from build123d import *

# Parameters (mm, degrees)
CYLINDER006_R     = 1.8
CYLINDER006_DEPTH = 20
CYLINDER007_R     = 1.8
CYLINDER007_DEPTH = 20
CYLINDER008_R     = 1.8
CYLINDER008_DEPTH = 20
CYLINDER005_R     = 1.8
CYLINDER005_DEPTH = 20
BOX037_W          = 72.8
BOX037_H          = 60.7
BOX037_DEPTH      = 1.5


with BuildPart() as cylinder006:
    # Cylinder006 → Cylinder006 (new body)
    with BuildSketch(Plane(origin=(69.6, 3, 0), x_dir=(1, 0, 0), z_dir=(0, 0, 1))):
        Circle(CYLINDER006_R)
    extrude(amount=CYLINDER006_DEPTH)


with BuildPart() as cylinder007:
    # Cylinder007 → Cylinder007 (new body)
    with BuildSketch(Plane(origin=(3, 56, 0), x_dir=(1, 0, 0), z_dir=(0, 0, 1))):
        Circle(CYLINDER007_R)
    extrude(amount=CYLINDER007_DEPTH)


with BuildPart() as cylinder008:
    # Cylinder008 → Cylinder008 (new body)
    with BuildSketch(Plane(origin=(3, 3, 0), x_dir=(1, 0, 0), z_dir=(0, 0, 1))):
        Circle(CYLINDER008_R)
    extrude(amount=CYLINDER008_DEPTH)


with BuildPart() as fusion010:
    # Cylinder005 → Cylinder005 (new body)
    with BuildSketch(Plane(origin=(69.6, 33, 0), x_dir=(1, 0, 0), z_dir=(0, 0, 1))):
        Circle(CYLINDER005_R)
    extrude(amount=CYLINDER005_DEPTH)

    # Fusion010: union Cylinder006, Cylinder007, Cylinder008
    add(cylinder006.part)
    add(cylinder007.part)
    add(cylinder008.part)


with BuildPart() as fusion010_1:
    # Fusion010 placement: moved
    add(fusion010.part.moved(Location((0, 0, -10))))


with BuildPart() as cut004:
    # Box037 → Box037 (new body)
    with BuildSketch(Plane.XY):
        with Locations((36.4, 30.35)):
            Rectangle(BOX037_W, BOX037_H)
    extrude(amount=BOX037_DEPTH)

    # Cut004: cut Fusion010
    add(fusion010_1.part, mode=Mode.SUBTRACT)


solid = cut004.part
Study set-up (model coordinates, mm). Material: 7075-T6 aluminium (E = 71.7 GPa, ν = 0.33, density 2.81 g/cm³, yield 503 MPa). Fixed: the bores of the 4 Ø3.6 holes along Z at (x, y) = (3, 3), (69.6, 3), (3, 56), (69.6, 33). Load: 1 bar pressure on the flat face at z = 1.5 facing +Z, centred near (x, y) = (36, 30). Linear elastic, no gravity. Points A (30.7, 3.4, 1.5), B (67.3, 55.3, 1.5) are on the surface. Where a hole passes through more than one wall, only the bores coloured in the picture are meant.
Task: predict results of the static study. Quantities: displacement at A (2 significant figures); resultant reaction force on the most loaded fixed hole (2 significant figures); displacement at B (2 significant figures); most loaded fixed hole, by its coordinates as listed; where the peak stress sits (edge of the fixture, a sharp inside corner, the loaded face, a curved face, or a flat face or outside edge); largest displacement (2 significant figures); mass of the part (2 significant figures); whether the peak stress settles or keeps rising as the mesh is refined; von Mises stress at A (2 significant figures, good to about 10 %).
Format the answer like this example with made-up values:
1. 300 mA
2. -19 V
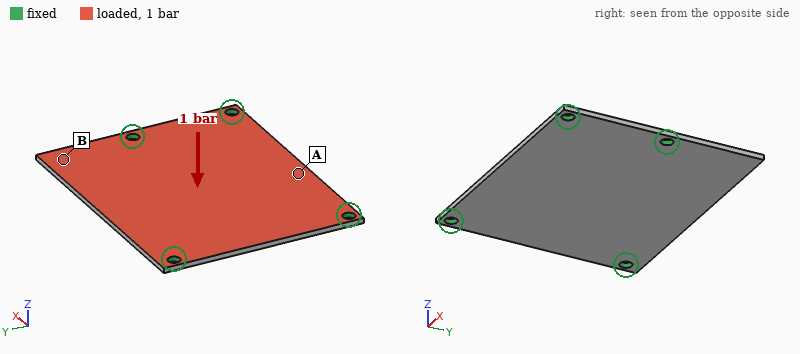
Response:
1. 0.29 mm
2. 170 N
3. 0.29 mm
4. (69.6, 33)
5. edge of the fixture
6. 0.57 mm
7. 18 g
8. keeps rising
9. 56 MPa
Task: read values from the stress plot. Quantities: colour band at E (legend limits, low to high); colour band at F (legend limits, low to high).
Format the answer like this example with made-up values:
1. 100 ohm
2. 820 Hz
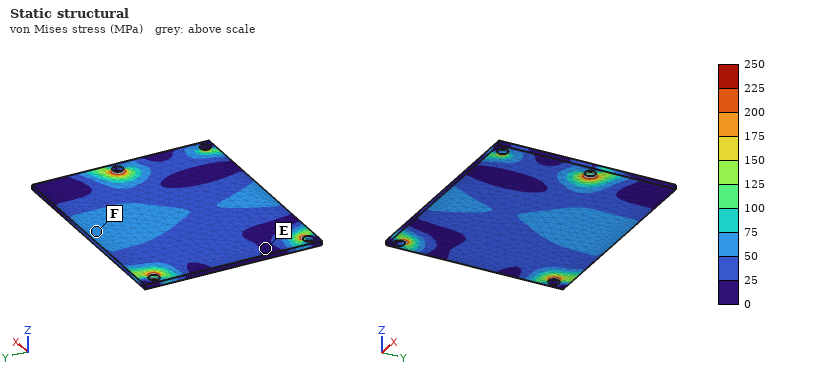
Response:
1. 0 to 25 MPa
2. 50 to 75 MPa
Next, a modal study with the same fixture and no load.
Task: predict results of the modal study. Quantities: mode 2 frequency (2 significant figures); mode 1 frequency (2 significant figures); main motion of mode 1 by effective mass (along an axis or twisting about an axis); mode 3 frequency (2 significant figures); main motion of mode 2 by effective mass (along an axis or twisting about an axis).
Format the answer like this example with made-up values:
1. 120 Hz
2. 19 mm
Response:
1. 1700 Hz
2. 1300 Hz
3. along Z
4. 2600 Hz
5. along Z
